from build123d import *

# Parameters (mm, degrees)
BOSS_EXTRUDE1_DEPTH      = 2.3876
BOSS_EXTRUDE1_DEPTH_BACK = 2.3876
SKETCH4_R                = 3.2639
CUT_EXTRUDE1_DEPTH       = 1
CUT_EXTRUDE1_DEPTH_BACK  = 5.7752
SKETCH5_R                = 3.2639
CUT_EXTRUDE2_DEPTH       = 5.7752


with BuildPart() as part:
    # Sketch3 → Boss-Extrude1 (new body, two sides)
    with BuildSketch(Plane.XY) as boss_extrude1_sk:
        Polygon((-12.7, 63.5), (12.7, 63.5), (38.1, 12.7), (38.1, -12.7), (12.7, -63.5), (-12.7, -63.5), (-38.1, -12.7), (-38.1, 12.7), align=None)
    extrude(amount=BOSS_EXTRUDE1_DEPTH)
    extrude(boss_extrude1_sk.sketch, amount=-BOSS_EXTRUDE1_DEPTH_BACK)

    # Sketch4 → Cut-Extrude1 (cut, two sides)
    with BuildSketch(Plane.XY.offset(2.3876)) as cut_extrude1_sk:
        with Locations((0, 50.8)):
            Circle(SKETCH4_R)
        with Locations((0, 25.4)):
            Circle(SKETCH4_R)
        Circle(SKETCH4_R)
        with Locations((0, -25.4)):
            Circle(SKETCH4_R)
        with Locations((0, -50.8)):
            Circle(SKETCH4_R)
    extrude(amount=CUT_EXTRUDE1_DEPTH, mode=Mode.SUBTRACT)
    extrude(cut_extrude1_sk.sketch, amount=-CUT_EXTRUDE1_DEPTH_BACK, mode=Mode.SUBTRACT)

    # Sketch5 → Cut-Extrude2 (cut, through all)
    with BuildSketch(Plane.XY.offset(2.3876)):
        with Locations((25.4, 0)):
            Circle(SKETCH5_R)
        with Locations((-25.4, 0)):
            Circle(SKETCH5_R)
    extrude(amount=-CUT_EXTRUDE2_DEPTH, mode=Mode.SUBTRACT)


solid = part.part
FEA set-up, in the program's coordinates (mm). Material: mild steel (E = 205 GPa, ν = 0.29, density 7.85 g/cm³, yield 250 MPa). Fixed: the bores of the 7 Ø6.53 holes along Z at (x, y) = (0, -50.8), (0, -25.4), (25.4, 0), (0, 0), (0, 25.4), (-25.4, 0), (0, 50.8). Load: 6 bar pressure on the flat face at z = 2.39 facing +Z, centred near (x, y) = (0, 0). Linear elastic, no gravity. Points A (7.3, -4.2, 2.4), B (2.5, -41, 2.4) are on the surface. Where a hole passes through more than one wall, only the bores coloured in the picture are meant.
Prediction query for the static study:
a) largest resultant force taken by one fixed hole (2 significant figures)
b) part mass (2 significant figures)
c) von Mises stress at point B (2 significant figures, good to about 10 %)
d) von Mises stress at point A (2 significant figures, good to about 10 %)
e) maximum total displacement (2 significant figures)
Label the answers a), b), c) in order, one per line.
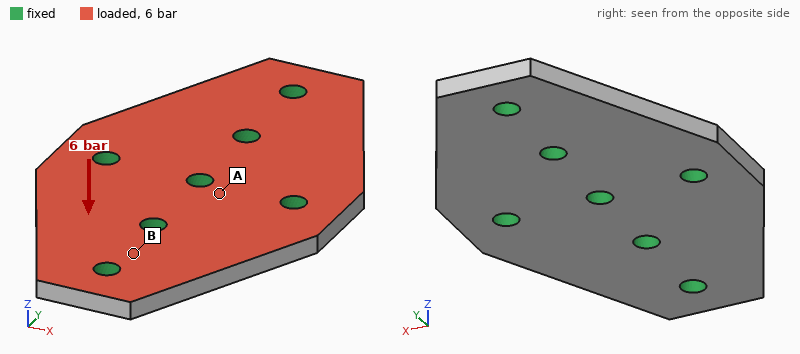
a) 690 N
b) 260 g
c) 18 MPa
d) 4.0 MPa
e) 9.0 µm
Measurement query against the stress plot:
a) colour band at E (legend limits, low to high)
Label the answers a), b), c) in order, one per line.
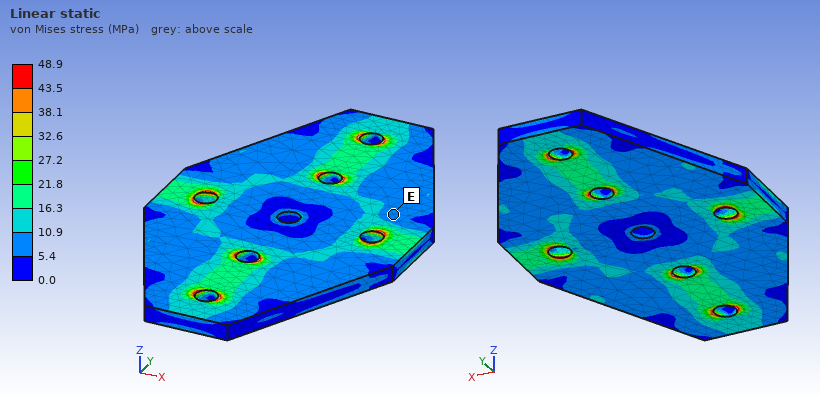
a) 5.4 to 10.9 MPa
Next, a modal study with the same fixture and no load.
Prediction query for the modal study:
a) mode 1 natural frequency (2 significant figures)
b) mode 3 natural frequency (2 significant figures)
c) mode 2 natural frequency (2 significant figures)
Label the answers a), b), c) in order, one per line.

a) 8300 Hz
b) 8800 Hz
c) 8600 Hz
